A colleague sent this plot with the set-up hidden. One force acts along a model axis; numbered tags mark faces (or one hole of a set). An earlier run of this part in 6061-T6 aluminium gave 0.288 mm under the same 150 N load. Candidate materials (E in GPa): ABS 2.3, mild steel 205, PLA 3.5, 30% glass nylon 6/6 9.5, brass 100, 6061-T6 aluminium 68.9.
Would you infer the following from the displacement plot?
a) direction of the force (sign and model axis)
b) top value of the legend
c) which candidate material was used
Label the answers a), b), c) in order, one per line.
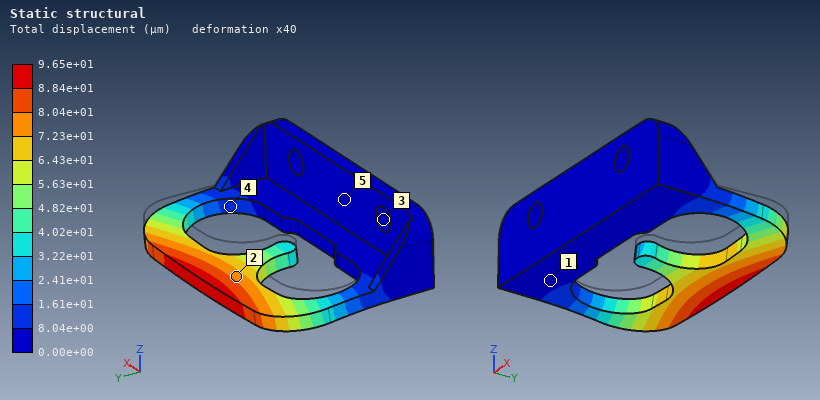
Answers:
a) -Z
b) 9.65e+01 µm
c) mild steel
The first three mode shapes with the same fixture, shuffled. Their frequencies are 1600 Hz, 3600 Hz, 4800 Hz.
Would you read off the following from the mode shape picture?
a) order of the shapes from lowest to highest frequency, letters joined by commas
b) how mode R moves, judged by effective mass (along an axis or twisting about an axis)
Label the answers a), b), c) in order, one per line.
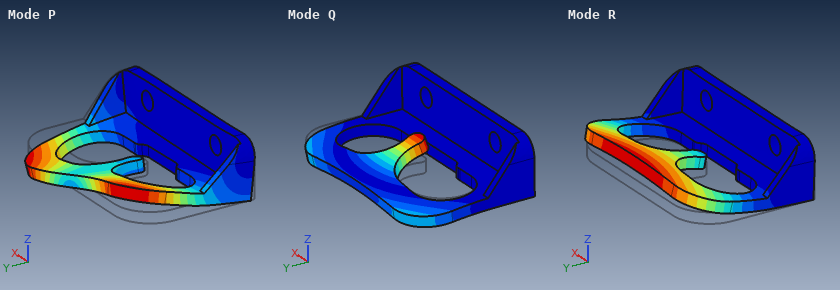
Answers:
a) R, P, Q
b) along Z
